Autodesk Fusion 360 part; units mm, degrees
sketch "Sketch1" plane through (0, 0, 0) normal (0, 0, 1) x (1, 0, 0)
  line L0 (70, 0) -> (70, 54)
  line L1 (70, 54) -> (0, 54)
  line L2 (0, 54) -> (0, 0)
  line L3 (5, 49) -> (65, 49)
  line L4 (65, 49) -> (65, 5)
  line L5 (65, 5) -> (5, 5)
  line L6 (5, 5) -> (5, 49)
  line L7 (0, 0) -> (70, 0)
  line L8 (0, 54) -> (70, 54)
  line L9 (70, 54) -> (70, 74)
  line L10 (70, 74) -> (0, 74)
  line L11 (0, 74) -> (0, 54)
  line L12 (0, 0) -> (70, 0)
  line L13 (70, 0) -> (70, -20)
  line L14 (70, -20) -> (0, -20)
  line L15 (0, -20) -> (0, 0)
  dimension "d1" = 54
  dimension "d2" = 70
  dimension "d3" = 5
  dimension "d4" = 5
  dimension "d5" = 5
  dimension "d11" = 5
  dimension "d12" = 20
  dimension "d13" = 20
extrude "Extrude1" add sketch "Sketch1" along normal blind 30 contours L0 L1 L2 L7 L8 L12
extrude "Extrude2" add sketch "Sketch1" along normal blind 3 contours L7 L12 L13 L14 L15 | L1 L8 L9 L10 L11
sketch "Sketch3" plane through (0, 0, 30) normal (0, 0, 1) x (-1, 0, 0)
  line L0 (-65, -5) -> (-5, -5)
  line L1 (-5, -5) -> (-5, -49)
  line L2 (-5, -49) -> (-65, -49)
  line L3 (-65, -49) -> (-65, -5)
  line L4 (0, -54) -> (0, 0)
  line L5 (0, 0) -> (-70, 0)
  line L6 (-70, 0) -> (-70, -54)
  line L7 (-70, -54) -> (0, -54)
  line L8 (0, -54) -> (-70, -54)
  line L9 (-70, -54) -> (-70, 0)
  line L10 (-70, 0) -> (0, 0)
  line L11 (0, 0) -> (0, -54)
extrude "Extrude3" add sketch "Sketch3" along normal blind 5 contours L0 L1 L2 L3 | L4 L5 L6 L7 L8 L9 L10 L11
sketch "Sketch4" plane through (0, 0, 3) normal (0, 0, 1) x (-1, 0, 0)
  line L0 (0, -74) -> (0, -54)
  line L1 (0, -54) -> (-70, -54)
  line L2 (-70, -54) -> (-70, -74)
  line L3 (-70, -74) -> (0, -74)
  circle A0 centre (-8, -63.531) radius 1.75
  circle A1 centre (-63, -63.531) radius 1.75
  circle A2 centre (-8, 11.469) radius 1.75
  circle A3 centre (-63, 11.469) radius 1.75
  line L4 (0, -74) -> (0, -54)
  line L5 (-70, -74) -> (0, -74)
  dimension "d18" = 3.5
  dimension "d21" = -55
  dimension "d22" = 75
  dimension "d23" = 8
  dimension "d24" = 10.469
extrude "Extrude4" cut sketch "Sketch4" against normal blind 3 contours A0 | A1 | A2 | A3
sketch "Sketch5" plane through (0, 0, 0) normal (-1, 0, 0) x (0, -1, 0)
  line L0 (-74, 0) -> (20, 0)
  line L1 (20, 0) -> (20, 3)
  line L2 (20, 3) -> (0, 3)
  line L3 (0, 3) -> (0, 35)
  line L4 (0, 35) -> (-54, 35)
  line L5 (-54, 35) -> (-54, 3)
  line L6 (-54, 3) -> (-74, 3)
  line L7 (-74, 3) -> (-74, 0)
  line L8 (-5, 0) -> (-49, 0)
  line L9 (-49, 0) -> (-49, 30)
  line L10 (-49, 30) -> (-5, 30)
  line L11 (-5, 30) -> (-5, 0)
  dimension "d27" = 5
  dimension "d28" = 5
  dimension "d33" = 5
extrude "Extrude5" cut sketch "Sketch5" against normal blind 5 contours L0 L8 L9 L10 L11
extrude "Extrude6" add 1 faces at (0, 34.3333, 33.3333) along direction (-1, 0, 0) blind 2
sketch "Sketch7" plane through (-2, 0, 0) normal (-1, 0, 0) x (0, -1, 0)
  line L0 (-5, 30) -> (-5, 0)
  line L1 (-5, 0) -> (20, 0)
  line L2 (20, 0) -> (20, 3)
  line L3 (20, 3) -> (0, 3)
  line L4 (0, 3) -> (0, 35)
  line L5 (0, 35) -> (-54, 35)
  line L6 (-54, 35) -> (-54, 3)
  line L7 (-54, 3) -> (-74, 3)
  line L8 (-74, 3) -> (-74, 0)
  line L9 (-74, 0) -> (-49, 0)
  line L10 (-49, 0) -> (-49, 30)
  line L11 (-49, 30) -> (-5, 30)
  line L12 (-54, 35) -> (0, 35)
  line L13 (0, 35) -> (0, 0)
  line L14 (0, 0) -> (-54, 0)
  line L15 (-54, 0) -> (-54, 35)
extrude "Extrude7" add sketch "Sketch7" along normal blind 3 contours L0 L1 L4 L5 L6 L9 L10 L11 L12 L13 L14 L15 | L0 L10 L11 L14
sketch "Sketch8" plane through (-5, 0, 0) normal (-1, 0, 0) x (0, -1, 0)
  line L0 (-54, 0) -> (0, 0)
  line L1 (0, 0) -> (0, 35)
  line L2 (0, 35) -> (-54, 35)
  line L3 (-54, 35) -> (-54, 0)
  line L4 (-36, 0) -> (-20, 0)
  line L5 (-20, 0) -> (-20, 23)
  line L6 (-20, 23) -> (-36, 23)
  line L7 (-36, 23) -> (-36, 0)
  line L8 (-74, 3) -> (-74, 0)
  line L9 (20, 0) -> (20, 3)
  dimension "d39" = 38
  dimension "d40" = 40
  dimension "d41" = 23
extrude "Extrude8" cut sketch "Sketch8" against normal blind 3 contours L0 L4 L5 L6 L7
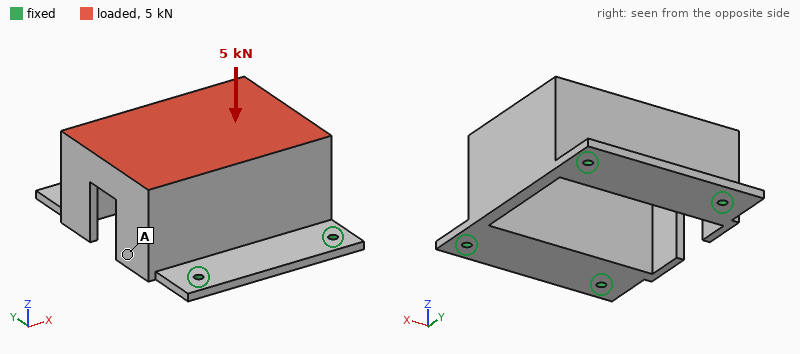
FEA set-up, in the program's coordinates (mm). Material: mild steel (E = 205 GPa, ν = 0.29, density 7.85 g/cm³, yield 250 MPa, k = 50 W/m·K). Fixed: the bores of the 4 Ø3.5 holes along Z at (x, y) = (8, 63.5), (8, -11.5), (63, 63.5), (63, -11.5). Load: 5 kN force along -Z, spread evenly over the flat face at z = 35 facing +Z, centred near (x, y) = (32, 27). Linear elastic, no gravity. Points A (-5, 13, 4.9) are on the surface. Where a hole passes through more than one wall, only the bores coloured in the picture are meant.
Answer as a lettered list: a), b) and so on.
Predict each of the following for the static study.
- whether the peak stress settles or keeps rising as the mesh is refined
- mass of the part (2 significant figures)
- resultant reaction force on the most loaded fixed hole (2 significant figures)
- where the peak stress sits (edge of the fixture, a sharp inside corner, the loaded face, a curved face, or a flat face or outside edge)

a) keeps rising
b) 480 g
c) 1.6 kN
d) edge of the fixture
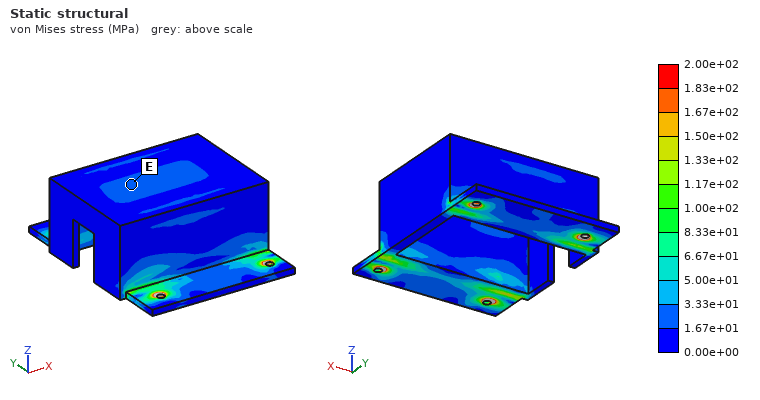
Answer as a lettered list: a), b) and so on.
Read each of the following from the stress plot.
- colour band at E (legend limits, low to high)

a) 1.67e+01 to 3.33e+01 MPa
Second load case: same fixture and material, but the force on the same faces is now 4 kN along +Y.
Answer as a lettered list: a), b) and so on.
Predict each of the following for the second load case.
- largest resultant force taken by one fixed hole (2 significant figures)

a) 1.5 kN
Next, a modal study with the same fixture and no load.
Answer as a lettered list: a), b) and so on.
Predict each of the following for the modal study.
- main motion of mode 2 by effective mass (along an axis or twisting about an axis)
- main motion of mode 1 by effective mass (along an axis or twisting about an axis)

a) along Z
b) along X
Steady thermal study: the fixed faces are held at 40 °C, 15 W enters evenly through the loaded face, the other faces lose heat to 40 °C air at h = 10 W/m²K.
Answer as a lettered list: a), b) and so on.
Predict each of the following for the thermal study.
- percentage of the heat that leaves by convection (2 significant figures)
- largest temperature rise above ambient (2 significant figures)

a) 23 %
b) 23 K
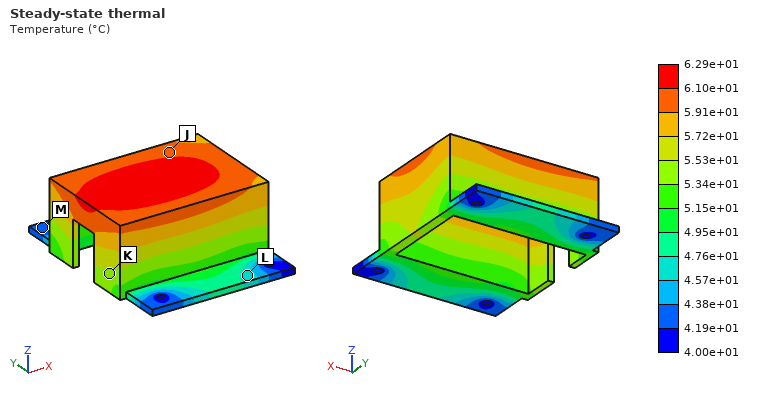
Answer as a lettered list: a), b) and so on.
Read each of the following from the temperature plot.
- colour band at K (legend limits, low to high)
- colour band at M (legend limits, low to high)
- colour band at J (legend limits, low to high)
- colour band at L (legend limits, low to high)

a) 5.34e+01 to 5.53e+01 °C
b) 4.19e+01 to 4.38e+01 °C
c) 5.91e+01 to 6.10e+01 °C
d) 4.57e+01 to 4.76e+01 °C
